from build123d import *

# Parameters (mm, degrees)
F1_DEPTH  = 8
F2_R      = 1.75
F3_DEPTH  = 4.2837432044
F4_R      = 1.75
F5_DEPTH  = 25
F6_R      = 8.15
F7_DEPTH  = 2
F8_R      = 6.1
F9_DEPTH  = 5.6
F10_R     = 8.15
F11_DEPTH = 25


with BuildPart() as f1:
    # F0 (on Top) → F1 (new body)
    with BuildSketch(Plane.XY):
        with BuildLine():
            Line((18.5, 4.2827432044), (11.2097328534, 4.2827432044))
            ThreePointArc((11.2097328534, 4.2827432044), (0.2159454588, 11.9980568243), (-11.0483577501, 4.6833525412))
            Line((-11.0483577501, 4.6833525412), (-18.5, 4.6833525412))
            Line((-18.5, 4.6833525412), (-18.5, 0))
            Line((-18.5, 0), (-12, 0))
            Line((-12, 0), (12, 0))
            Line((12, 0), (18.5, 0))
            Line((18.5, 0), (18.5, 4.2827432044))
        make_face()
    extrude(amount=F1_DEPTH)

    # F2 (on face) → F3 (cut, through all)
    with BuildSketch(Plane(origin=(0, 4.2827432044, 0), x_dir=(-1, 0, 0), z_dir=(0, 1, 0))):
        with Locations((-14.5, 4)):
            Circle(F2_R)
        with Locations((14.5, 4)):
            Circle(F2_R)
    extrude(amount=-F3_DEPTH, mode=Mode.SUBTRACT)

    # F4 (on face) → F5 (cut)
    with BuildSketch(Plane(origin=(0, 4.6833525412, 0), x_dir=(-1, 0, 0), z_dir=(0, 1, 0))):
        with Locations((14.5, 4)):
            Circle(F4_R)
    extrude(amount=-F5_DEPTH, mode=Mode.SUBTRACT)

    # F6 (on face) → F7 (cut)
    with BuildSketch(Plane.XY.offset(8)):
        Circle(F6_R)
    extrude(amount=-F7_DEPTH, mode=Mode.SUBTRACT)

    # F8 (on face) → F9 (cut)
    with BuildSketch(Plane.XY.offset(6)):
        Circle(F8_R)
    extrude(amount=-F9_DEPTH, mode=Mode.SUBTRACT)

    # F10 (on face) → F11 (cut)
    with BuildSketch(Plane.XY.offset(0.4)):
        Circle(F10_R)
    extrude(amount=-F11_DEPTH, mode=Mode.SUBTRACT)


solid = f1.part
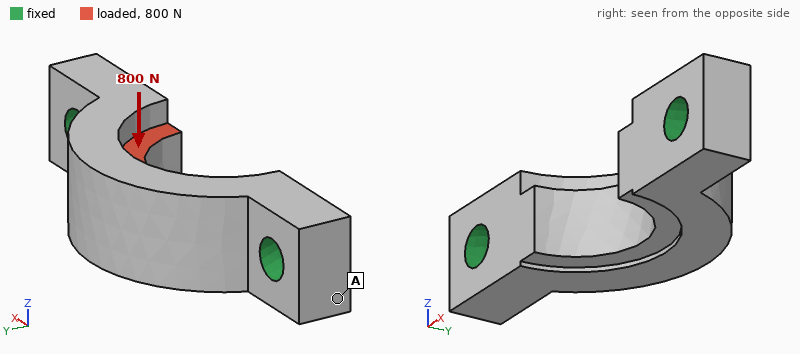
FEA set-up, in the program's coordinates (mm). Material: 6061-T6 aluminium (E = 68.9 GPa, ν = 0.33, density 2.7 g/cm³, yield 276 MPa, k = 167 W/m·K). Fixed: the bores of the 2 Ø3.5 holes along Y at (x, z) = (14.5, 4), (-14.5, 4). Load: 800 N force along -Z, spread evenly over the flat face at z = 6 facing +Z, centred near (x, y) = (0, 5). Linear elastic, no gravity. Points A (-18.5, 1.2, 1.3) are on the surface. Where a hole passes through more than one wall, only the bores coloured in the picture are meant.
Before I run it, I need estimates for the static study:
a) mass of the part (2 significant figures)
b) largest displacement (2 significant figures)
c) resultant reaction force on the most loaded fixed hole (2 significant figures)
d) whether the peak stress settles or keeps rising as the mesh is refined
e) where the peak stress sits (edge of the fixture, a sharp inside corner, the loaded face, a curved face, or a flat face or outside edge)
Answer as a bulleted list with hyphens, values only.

- 4.4 g
- 19 µm
- 410 N
- keeps rising
- edge of the fixture
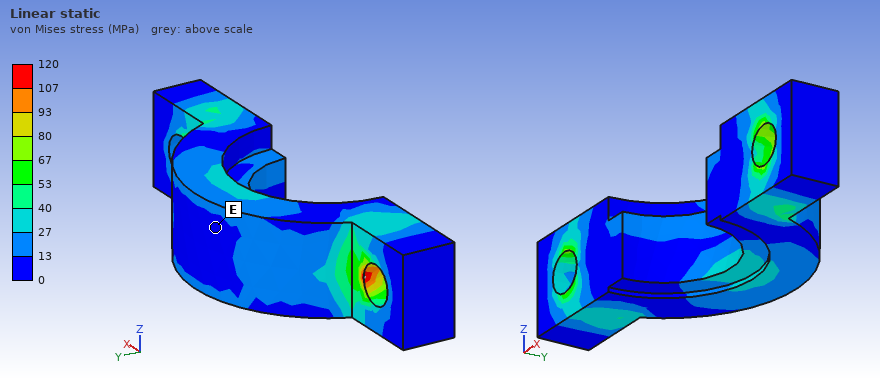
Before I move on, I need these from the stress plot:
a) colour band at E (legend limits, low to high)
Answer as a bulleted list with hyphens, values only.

- 0 to 13 MPa
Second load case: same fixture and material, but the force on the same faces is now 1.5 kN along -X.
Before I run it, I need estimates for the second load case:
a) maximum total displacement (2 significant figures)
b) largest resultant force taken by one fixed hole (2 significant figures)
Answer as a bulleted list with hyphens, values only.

- 7.2 µm
- 780 N
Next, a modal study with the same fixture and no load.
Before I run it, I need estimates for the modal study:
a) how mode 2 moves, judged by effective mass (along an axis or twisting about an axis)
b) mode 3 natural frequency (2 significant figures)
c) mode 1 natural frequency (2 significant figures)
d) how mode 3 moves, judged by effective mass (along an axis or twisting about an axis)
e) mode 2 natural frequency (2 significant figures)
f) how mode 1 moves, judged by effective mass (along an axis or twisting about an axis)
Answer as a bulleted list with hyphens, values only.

- along Y
- 49 kHz
- 19 kHz
- along X
- 39 kHz
- along Z
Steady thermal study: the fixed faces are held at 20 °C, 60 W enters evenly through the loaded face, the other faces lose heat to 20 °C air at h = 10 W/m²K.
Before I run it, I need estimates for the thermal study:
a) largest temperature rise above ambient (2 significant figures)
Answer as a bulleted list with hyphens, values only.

- 53 K
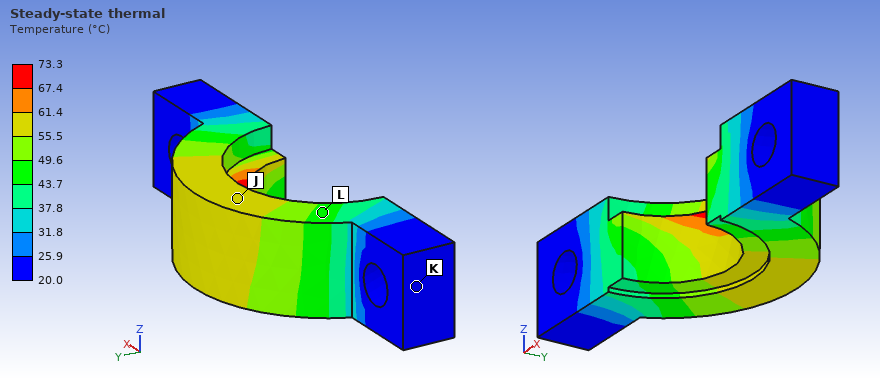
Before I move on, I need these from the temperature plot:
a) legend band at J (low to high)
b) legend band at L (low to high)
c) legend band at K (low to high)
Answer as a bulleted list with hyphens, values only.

- 55.5 to 61.4 °C
- 43.7 to 49.6 °C
- 20.0 to 25.9 °C
